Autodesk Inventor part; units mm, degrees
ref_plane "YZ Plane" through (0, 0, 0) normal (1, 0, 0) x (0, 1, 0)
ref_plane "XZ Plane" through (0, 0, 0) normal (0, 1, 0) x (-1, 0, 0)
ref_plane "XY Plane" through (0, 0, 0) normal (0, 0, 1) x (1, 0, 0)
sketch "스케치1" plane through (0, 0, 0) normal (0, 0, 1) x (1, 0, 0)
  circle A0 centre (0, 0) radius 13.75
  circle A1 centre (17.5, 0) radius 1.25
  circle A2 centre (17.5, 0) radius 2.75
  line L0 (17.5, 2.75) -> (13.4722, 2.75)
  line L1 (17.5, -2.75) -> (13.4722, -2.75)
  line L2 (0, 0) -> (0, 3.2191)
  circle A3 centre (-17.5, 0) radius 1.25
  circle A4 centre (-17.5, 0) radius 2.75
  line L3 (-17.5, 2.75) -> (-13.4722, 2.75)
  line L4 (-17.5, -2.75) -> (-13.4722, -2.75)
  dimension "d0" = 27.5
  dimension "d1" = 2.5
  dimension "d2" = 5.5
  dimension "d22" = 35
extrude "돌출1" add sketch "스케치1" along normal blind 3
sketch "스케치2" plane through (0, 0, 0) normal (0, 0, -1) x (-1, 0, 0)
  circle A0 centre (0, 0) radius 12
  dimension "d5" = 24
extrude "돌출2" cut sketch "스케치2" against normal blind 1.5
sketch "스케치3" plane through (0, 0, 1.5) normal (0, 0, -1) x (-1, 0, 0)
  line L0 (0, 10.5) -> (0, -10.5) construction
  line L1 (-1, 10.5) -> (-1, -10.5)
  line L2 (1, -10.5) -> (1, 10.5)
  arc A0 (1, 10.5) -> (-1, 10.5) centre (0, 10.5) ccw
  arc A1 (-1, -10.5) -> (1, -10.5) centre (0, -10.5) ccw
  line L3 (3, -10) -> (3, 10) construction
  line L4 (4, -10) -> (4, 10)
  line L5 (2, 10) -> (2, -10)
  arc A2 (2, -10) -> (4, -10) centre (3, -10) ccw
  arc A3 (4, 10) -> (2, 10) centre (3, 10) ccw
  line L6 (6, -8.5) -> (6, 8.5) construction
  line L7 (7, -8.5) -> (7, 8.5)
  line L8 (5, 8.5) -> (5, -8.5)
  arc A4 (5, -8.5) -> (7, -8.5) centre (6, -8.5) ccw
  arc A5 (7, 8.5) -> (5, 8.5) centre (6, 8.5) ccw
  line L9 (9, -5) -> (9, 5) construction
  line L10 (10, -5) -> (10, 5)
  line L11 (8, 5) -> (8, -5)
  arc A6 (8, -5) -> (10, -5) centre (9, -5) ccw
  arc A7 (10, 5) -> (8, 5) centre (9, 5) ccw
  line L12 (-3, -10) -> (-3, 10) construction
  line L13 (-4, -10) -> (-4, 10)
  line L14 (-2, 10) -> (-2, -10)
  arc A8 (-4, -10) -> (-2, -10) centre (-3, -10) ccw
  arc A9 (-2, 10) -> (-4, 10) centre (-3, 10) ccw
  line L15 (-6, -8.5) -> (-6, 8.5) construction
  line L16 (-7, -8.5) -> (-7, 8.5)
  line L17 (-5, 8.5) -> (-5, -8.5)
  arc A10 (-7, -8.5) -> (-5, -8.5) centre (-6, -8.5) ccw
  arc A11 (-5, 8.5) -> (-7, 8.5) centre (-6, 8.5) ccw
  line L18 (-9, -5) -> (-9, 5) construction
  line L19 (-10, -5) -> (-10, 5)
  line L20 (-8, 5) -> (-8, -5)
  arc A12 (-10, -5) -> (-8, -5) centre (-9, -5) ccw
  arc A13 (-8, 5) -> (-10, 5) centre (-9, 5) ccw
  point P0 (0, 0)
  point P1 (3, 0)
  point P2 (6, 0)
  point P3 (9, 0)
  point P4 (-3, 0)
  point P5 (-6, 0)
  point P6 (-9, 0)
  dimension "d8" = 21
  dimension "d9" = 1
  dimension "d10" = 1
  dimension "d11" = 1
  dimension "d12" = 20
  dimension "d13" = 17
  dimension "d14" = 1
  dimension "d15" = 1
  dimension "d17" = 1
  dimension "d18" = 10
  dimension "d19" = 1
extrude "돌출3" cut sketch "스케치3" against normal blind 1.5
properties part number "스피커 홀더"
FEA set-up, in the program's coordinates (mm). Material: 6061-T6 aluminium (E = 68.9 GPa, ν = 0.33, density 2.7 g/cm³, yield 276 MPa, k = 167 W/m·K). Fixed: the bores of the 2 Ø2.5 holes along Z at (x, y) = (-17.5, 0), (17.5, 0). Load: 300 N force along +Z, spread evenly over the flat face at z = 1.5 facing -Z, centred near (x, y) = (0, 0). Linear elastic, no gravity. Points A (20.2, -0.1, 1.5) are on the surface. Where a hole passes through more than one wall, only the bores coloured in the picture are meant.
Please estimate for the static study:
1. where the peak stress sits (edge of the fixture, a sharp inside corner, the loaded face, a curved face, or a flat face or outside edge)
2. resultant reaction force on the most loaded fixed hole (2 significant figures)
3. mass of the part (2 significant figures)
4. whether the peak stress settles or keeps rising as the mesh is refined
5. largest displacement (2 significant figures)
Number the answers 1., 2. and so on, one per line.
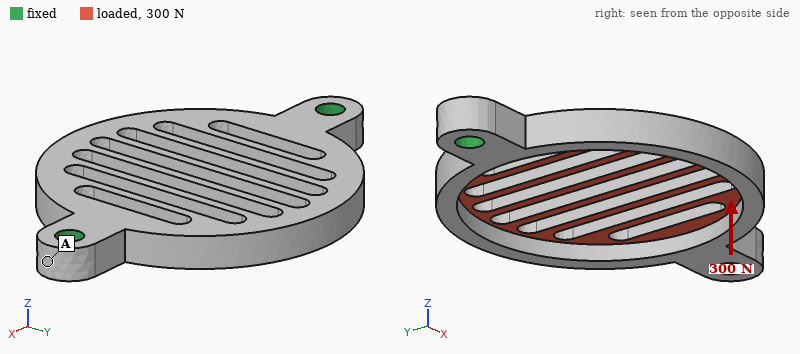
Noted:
1. edge of the fixture
2. 150 N
3. 2.4 g
4. keeps rising
5. 0.16 mm
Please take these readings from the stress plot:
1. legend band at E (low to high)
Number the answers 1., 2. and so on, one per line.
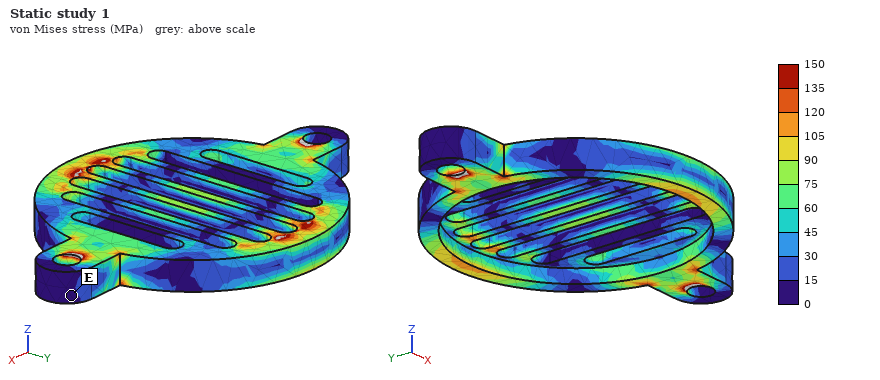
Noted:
1. 0 to 15 MPa
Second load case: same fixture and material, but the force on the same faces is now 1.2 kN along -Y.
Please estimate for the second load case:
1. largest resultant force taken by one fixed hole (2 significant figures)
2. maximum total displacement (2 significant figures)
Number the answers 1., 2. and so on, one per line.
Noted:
1. 600 N
2. 38 µm
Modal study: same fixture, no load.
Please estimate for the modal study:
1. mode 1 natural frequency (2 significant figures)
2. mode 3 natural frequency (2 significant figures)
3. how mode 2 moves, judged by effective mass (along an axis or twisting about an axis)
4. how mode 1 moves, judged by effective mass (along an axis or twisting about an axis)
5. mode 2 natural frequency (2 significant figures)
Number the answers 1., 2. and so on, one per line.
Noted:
1. 6200 Hz
2. 10 kHz
3. along Z
4. twisting about X
5. 7100 Hz
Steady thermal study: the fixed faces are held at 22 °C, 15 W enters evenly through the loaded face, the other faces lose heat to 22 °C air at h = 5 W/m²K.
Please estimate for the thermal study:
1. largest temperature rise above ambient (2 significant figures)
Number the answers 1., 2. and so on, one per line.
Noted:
1. 61 K
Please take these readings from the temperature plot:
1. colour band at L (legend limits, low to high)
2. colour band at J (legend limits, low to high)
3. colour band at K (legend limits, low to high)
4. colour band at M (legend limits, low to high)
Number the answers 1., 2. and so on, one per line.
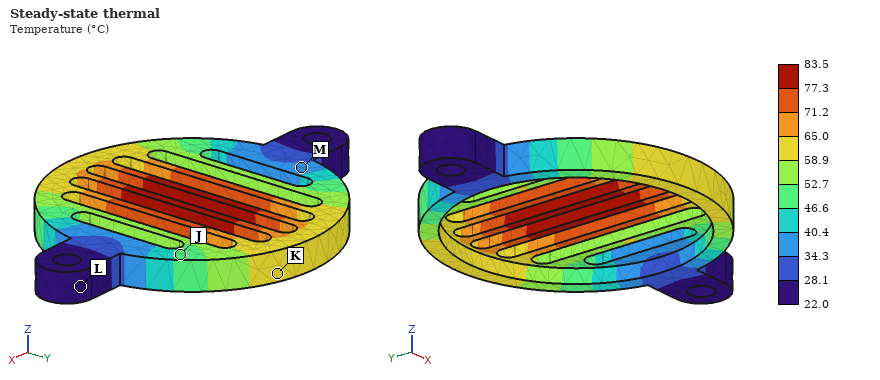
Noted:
1. 22.0 to 28.1 °C
2. 46.6 to 52.7 °C
3. 58.9 to 65.0 °C
4. 34.3 to 40.4 °C
